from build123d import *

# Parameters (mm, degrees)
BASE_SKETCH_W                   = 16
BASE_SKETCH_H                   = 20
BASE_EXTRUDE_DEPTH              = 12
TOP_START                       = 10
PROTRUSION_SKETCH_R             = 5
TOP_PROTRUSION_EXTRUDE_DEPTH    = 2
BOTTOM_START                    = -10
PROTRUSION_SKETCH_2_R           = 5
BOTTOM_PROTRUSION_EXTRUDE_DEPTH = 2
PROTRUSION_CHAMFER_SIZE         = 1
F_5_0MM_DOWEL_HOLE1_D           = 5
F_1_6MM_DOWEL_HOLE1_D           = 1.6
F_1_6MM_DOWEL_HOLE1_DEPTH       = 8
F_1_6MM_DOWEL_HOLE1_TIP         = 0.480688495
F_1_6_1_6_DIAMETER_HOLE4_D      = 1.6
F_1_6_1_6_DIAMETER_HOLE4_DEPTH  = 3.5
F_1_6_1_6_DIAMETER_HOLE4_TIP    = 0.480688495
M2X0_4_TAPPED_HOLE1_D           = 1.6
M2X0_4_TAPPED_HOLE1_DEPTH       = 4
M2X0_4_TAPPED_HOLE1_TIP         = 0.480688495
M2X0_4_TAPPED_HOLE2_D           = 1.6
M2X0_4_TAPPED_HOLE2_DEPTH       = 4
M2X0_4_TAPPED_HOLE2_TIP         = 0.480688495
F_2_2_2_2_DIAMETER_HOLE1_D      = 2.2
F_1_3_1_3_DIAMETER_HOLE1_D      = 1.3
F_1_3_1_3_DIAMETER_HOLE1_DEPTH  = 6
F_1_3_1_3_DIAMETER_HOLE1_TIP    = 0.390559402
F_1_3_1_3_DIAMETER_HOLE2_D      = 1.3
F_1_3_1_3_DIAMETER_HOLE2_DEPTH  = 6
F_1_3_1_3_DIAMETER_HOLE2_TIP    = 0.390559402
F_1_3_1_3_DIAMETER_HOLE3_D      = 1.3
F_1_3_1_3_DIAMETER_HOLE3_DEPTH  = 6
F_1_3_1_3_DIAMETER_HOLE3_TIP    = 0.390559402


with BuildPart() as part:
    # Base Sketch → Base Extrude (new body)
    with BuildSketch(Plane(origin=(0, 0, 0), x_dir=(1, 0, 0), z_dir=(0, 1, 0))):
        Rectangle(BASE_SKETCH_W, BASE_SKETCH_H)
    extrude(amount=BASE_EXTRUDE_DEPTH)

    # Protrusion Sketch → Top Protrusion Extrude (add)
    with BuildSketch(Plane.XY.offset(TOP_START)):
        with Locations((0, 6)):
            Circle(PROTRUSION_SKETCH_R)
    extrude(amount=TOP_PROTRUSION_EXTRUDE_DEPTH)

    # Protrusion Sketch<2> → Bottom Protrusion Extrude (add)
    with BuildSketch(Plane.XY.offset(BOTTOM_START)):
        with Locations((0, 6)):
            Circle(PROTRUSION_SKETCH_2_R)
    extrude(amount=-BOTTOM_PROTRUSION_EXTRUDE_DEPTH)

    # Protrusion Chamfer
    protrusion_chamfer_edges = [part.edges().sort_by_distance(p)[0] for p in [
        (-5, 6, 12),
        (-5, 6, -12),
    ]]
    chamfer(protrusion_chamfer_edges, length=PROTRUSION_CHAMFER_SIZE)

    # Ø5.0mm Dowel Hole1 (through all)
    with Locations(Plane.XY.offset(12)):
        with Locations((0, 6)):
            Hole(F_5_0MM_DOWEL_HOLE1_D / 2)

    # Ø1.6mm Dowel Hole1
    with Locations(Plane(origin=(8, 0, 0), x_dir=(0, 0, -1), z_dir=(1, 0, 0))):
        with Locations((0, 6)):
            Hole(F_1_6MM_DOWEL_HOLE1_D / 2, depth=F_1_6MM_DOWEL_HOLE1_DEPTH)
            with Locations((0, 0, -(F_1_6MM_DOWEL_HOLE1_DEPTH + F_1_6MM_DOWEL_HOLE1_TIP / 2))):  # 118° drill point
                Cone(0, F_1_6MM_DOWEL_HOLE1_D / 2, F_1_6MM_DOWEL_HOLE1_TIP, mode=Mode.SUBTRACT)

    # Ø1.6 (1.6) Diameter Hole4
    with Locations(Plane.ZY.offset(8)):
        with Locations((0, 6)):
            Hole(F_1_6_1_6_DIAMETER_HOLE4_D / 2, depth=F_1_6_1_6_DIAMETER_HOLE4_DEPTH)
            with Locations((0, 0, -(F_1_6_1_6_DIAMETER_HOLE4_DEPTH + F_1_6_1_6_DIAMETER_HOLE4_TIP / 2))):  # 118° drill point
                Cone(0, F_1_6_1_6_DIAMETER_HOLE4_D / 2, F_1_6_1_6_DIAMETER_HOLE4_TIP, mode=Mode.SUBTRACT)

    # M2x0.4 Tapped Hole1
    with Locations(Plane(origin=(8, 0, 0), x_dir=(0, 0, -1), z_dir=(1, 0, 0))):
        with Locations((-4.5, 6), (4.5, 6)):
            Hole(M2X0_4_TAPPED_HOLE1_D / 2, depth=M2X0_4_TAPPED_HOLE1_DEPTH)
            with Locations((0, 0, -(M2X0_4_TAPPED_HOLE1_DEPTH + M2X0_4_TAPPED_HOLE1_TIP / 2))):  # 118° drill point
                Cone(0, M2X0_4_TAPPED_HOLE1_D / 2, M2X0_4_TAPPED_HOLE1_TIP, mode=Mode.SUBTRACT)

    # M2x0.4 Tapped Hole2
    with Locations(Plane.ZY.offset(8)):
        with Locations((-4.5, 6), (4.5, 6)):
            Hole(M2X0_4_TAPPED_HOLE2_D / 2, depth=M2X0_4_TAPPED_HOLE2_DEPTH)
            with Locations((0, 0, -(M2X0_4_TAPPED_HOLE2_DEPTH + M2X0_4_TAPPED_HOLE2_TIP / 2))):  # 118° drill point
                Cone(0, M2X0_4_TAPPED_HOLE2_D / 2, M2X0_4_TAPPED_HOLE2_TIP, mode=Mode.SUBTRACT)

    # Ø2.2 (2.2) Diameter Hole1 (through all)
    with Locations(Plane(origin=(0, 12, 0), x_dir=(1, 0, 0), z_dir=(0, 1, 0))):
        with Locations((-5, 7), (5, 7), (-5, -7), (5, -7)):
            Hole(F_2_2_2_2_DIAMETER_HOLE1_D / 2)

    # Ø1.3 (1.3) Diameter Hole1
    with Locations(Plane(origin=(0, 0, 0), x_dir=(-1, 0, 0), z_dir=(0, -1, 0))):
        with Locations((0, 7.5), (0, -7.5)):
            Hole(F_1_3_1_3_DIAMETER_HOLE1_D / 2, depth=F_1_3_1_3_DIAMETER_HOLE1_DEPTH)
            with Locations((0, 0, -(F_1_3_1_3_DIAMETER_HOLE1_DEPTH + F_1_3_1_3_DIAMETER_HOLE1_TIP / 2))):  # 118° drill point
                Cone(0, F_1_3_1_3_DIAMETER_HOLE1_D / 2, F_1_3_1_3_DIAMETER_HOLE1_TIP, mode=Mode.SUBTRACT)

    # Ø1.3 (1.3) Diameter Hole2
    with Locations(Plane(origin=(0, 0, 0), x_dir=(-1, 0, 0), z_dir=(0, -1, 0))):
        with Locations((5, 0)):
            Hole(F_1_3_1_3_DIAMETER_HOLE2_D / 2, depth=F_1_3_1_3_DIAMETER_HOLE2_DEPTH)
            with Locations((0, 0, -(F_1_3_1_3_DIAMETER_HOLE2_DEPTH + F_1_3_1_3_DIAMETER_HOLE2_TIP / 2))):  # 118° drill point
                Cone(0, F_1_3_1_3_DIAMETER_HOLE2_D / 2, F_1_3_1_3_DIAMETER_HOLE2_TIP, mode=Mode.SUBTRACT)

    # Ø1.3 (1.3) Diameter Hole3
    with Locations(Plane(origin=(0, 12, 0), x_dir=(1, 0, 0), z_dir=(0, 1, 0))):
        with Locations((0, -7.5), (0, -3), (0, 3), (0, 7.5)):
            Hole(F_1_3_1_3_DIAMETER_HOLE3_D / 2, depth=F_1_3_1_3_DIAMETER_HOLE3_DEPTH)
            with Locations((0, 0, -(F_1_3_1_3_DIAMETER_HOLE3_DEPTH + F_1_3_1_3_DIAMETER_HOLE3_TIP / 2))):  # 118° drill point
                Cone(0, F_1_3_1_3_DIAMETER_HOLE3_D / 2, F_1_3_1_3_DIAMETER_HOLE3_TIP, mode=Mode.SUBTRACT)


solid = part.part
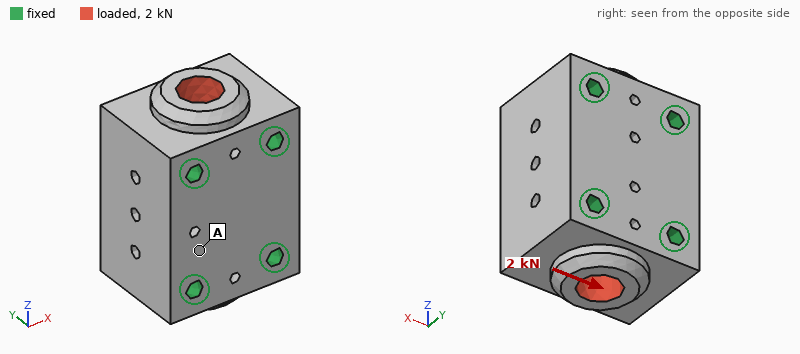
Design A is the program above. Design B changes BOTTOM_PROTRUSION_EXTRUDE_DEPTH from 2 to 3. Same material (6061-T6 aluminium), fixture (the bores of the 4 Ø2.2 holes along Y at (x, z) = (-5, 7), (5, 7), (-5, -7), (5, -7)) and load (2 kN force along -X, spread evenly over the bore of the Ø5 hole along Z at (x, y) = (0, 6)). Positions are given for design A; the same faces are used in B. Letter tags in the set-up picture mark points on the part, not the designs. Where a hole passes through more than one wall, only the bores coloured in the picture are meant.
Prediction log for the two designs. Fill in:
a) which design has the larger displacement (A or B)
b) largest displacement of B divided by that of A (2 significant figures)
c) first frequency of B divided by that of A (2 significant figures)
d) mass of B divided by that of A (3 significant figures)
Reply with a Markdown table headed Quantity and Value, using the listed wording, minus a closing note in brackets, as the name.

| Quantity | Value |
|---|---|
| which design has the larger displacement | B |
| largest displacement of B divided by that of A | 1.4 |
| first frequency of B divided by that of A | 1.0 |
| mass of B divided by that of A | 1.02 |
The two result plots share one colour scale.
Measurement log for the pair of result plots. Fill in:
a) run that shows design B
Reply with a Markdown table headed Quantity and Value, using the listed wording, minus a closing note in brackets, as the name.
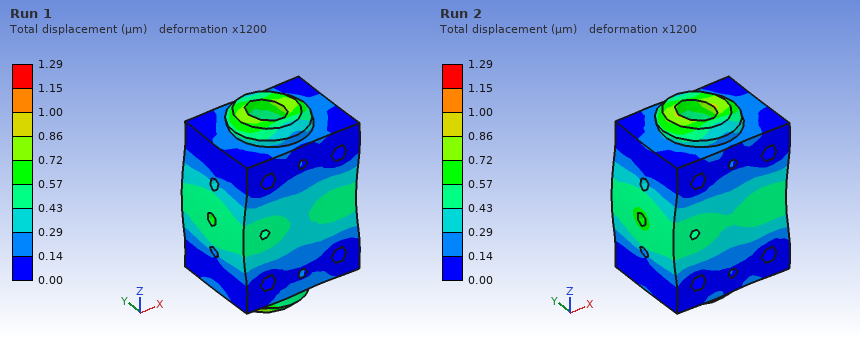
| Quantity | Value |
|---|---|
| run that shows design B | Run 1 |
